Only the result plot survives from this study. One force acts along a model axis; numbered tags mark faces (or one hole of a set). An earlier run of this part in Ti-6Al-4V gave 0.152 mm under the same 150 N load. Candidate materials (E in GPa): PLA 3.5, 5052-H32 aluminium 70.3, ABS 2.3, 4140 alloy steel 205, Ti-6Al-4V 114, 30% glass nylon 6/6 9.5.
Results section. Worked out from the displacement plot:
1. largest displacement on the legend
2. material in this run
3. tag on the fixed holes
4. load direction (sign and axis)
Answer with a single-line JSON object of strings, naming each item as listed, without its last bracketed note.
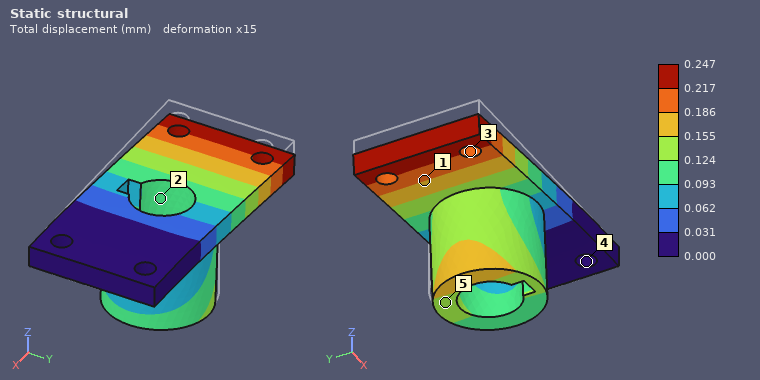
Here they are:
{"largest displacement on the legend": "0.247 mm", "material in this run": "5052-H32 aluminium", "tag on the fixed holes": "4", "load direction": "-Z"}
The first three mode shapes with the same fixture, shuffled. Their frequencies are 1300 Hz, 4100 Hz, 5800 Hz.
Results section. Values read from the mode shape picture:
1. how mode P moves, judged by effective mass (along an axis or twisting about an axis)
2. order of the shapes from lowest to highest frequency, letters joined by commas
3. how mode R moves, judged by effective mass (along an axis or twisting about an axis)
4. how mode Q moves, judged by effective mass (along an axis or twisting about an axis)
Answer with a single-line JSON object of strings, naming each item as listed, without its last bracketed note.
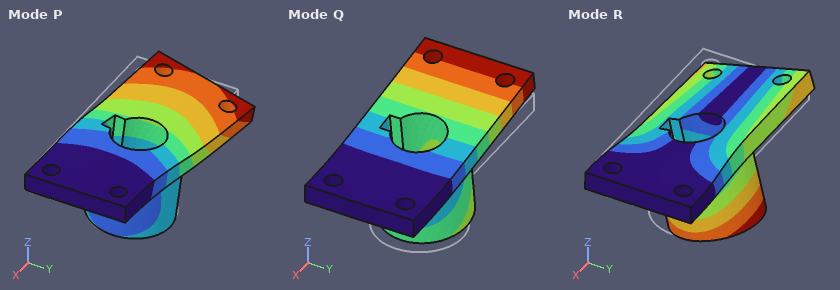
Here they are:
{"how mode P moves, judged by effective mass": "along Y", "order of the shapes from lowest to highest frequency, letters joined by commas": "Q, R, P", "how mode R moves, judged by effective mass": "along Y", "how mode Q moves, judged by effective mass": "along Z"}
